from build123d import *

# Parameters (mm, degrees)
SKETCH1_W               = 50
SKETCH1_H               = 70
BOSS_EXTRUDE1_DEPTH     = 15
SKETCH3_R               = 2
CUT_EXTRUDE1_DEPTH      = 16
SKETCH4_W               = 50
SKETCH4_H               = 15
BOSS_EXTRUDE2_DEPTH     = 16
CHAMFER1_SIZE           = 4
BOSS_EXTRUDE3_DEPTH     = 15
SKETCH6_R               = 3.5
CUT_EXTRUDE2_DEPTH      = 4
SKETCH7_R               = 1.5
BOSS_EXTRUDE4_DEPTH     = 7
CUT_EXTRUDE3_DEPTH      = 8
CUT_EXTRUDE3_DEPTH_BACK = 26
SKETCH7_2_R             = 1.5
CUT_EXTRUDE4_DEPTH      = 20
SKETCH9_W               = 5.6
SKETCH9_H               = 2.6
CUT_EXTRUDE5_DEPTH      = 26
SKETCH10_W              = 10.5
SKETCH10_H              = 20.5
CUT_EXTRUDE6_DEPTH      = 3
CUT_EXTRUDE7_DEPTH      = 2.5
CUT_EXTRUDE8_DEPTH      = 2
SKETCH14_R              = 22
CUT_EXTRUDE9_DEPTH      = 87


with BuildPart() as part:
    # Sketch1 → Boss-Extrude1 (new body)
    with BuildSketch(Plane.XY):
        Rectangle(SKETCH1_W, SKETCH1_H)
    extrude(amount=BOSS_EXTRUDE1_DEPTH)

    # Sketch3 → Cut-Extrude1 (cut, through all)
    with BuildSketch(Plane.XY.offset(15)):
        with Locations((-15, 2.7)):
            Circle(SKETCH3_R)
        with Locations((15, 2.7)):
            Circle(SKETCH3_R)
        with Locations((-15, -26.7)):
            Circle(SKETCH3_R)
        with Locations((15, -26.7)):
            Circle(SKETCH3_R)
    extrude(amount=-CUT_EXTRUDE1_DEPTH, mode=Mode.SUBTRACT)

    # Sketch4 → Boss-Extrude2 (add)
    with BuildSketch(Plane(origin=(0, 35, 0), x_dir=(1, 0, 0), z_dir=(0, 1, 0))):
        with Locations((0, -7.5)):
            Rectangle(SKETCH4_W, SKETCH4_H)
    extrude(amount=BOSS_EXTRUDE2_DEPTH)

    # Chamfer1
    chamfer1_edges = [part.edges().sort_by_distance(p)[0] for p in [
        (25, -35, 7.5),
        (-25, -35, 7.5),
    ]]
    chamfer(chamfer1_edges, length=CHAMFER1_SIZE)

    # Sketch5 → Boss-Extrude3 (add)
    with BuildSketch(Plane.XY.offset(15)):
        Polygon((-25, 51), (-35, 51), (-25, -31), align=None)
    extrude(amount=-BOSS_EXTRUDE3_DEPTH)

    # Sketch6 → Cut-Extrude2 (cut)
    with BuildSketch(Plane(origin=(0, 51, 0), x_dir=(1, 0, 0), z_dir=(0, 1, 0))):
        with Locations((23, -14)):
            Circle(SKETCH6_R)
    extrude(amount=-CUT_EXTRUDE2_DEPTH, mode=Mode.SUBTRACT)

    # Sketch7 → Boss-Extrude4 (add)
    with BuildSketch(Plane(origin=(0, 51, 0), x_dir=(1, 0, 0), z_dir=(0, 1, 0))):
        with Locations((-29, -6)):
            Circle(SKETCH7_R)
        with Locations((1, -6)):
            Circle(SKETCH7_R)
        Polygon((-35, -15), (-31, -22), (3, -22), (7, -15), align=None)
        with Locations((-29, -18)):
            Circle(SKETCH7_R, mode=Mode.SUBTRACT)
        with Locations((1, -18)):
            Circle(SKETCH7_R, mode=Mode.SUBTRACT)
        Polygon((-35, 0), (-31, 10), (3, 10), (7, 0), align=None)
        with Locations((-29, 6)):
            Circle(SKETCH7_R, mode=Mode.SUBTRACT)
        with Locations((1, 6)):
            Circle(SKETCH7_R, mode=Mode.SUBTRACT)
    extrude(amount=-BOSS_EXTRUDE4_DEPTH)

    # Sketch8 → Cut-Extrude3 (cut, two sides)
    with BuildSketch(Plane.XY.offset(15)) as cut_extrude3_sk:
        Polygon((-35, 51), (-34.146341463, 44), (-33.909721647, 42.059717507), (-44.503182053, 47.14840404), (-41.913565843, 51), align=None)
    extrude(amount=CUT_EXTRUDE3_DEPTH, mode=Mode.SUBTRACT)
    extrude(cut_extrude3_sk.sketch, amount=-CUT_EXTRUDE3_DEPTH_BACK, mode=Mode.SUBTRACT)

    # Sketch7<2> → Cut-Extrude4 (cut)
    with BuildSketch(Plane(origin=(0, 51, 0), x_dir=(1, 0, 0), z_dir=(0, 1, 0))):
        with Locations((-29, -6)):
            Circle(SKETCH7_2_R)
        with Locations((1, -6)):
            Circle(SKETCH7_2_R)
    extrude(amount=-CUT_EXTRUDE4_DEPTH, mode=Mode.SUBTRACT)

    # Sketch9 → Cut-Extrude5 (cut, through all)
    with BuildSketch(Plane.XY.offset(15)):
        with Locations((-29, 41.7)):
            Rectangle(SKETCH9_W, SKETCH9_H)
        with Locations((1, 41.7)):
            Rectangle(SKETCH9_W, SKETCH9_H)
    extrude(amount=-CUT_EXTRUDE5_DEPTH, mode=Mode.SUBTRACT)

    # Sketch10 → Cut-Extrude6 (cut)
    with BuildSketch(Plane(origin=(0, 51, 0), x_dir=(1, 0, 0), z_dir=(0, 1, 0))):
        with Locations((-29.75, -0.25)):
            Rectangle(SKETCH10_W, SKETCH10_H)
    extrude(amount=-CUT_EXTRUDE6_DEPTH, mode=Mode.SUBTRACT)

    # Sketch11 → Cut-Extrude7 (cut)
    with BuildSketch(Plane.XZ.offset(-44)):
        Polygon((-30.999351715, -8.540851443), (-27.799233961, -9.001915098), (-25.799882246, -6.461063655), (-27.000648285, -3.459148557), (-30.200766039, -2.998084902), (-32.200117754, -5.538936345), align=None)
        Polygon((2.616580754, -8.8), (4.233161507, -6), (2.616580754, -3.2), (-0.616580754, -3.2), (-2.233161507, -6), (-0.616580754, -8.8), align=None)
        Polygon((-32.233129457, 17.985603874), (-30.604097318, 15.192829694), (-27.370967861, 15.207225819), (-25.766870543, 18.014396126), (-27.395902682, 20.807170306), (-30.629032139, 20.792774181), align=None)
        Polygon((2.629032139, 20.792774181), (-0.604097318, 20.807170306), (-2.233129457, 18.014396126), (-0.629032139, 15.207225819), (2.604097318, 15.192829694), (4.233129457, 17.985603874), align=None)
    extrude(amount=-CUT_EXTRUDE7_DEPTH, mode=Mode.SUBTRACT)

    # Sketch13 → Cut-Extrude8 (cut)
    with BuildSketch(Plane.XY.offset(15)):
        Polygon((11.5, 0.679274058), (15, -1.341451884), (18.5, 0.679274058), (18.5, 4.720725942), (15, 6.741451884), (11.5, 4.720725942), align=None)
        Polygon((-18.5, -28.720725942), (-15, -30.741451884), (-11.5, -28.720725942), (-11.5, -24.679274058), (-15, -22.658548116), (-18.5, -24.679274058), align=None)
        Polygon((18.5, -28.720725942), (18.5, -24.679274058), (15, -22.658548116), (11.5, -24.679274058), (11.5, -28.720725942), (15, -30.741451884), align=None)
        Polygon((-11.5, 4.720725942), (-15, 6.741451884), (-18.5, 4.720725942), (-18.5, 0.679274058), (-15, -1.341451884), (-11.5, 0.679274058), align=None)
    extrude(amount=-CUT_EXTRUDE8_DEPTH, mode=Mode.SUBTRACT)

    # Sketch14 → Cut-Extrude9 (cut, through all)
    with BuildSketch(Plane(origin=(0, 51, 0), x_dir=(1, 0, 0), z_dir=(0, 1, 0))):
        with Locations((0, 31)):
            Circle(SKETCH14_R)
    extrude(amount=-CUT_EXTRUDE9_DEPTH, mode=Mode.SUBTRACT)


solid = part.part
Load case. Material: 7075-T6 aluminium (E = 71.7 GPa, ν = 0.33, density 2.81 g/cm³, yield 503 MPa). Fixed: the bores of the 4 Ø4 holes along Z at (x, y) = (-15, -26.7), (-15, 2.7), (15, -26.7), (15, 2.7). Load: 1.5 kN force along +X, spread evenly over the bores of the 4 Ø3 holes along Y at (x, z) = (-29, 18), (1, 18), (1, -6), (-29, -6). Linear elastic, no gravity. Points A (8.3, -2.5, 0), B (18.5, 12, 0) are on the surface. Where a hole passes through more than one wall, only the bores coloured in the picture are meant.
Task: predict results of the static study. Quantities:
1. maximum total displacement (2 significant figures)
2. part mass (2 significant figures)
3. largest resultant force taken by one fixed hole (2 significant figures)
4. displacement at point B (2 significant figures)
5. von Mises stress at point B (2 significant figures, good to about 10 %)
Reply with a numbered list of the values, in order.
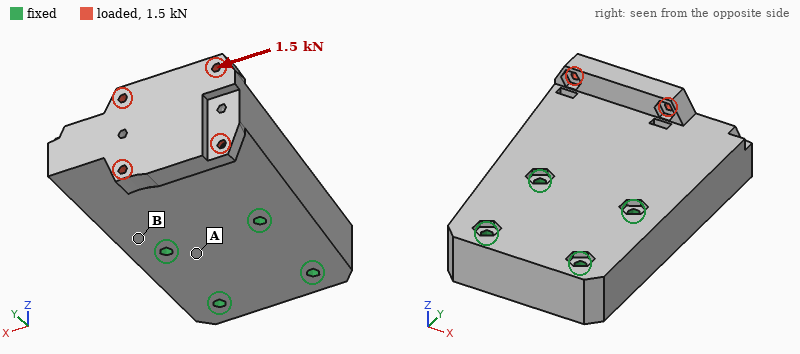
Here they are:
1. 13 µm
2. 200 g
3. 1.8 kN
4. 2.1 µm
5. 6.4 MPa
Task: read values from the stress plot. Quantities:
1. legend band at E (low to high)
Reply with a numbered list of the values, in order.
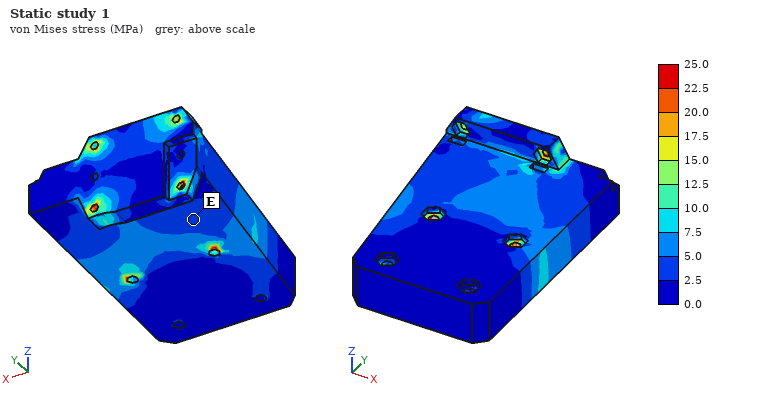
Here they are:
1. 2.5 to 5.0 MPa
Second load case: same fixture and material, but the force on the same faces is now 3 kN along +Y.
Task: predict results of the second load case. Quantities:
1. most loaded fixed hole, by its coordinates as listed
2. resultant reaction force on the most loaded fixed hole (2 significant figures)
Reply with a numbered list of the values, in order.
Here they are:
1. (-15, 2.7)
2. 1.9 kN
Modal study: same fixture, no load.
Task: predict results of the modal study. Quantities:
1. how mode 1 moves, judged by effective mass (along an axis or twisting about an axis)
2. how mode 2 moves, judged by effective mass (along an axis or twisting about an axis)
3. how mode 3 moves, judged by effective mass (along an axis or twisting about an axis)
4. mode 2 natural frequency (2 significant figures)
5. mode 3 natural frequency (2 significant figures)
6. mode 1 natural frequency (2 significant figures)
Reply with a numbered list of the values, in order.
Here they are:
1. along Z
2. twisting about Y
3. along X
4. 7500 Hz
5. 8600 Hz
6. 3700 Hz
